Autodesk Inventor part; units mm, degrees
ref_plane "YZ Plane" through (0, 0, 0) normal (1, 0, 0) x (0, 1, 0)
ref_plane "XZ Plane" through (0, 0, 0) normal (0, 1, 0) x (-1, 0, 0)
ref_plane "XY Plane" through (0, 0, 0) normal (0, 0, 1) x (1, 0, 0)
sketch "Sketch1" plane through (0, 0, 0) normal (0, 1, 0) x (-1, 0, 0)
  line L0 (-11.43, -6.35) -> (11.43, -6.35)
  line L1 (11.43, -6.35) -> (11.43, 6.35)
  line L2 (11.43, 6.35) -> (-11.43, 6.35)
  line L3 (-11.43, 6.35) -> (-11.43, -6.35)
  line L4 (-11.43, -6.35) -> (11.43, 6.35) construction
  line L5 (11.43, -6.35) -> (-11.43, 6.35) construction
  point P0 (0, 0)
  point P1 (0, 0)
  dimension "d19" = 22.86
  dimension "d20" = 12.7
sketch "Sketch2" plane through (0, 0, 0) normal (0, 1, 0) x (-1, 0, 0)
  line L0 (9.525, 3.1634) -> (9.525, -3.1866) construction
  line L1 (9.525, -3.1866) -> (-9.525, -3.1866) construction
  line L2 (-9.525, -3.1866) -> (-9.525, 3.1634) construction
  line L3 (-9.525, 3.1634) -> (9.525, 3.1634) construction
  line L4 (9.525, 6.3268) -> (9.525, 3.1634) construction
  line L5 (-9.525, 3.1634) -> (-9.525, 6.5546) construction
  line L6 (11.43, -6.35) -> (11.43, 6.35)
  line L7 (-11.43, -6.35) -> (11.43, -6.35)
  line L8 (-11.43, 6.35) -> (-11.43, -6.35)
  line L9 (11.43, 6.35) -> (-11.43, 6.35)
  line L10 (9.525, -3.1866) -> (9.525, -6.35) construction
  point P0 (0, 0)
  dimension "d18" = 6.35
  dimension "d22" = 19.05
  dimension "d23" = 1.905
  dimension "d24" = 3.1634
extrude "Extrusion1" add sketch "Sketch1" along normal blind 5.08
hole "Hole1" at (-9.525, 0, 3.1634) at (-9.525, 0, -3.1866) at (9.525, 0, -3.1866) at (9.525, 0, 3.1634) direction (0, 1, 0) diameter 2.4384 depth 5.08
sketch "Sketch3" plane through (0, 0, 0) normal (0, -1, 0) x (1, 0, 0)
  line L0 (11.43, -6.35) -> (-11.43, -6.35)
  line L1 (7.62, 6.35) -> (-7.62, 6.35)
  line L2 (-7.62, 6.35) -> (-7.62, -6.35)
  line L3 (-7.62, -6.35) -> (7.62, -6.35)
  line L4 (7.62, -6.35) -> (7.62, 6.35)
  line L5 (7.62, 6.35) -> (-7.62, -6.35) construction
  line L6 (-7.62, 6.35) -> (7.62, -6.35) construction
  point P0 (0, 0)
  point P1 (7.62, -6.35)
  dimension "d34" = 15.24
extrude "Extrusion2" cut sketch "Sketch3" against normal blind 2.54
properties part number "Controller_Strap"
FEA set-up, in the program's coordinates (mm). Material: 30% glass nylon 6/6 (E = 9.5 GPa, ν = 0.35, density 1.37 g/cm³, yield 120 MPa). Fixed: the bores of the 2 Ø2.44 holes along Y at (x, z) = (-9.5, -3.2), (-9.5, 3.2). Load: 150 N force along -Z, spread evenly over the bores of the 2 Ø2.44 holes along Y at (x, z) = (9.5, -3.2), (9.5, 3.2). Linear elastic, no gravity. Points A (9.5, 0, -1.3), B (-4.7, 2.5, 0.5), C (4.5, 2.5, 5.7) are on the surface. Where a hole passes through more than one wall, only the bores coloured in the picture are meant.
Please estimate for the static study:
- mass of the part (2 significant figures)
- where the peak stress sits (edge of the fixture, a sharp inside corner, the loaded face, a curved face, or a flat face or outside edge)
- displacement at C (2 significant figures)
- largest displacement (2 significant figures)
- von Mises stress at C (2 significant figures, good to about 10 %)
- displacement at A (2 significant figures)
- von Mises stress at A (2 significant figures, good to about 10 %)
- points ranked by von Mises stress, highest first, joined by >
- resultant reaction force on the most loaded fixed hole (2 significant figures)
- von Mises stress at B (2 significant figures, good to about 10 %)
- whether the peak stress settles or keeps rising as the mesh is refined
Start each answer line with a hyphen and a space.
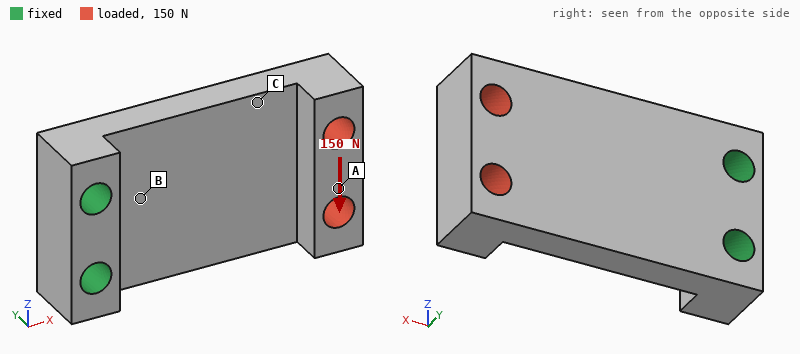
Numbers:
- 1.2 g
- edge of the fixture
- 0.11 mm
- 0.20 mm
- 16 MPa
- 0.16 mm
- 7.2 MPa
- B > C > A
- 340 N
- 25 MPa
- keeps rising
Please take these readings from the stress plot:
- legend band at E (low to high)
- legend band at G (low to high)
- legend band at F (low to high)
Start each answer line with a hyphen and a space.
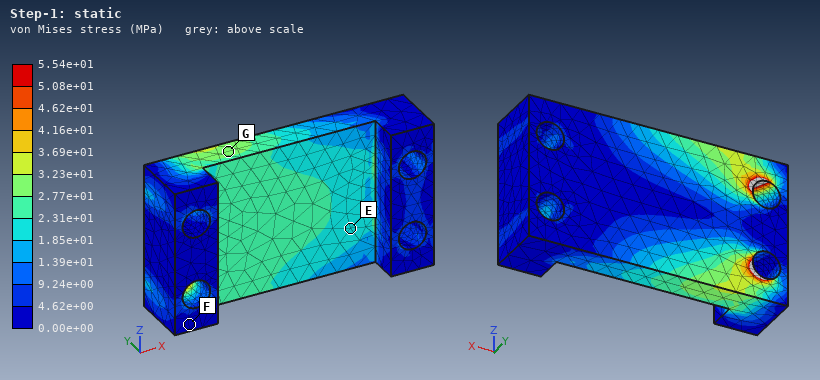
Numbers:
- 1.85e+01 to 2.31e+01 MPa
- 2.77e+01 to 3.23e+01 MPa
- 0.00e+00 to 4.62e+00 MPa
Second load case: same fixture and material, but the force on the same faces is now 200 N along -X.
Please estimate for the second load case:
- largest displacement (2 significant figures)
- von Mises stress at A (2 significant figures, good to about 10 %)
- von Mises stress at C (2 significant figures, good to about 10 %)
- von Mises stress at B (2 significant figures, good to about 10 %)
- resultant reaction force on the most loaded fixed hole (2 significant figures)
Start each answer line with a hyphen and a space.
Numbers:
- 0.31 mm
- 5.3 MPa
- 24 MPa
- 23 MPa
- 100 N
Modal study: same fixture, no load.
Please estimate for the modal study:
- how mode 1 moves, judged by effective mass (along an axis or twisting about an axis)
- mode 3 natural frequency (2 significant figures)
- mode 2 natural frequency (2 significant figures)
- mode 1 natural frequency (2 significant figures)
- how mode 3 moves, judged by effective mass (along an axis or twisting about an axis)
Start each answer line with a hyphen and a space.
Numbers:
- along Y
- 9000 Hz
- 7000 Hz
- 2300 Hz
- along Z
